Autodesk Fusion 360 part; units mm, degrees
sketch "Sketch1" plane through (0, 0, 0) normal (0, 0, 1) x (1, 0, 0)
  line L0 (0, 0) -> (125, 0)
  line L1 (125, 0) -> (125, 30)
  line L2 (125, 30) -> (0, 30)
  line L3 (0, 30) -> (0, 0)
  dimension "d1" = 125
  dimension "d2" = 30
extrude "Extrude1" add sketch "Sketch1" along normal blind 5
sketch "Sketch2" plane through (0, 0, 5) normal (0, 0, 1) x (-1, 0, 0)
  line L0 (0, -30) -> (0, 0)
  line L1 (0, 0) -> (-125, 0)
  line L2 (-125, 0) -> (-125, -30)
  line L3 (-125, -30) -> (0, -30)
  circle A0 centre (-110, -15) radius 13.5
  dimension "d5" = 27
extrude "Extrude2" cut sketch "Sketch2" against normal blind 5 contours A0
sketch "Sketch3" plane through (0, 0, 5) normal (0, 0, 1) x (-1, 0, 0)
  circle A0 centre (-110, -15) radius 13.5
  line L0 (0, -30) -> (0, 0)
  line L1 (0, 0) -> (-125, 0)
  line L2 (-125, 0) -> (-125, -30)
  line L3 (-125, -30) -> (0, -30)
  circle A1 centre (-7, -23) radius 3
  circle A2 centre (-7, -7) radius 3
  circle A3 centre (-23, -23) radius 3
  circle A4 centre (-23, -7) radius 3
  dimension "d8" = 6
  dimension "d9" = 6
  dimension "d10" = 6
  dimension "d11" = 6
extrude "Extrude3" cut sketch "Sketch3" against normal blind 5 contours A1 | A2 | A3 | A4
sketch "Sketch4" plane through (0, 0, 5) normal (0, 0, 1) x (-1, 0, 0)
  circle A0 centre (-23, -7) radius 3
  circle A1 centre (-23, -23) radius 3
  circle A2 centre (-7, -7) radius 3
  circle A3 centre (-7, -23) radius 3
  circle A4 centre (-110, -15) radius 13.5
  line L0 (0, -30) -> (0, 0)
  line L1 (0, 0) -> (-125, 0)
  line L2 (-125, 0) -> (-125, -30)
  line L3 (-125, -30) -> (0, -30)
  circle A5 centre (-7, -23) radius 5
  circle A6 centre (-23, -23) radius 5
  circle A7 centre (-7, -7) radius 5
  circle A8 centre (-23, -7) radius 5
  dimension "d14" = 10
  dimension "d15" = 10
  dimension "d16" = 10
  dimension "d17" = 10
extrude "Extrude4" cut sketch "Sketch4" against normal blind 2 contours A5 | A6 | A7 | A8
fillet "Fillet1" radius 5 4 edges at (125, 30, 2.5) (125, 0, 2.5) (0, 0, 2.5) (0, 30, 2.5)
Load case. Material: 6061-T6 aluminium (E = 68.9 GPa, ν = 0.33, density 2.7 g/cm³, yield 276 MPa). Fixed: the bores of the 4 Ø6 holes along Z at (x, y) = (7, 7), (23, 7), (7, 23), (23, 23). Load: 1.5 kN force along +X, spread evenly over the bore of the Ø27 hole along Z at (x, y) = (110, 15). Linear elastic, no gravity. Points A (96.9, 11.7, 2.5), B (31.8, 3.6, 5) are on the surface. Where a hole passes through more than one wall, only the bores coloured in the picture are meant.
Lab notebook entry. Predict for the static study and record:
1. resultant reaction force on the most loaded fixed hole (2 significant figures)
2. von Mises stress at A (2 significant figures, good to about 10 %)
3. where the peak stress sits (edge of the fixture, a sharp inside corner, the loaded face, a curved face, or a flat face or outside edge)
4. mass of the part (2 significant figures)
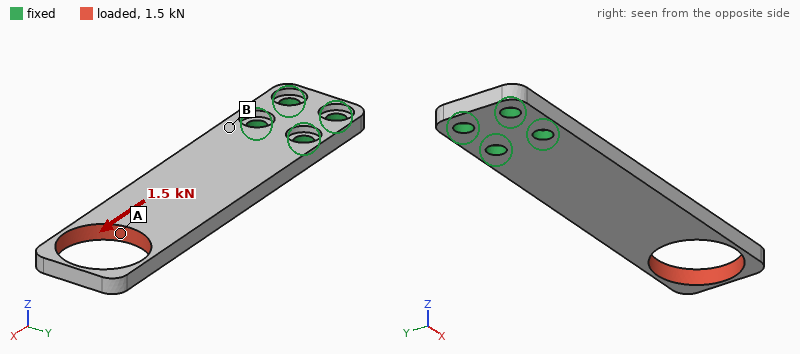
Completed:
660 N
31 MPa
the loaded face
40 g
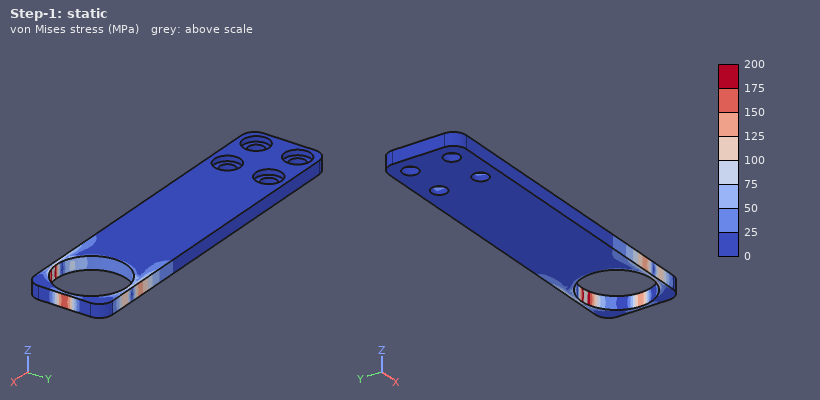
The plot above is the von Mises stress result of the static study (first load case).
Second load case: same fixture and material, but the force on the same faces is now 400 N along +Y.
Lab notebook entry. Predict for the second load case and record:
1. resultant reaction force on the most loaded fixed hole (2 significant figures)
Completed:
1.5 kN
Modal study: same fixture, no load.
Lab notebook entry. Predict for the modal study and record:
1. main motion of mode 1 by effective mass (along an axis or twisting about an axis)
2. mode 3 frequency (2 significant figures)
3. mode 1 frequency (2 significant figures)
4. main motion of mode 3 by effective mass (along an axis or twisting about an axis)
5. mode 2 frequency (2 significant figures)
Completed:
along Z
2600 Hz
520 Hz
along Y
2400 Hz
